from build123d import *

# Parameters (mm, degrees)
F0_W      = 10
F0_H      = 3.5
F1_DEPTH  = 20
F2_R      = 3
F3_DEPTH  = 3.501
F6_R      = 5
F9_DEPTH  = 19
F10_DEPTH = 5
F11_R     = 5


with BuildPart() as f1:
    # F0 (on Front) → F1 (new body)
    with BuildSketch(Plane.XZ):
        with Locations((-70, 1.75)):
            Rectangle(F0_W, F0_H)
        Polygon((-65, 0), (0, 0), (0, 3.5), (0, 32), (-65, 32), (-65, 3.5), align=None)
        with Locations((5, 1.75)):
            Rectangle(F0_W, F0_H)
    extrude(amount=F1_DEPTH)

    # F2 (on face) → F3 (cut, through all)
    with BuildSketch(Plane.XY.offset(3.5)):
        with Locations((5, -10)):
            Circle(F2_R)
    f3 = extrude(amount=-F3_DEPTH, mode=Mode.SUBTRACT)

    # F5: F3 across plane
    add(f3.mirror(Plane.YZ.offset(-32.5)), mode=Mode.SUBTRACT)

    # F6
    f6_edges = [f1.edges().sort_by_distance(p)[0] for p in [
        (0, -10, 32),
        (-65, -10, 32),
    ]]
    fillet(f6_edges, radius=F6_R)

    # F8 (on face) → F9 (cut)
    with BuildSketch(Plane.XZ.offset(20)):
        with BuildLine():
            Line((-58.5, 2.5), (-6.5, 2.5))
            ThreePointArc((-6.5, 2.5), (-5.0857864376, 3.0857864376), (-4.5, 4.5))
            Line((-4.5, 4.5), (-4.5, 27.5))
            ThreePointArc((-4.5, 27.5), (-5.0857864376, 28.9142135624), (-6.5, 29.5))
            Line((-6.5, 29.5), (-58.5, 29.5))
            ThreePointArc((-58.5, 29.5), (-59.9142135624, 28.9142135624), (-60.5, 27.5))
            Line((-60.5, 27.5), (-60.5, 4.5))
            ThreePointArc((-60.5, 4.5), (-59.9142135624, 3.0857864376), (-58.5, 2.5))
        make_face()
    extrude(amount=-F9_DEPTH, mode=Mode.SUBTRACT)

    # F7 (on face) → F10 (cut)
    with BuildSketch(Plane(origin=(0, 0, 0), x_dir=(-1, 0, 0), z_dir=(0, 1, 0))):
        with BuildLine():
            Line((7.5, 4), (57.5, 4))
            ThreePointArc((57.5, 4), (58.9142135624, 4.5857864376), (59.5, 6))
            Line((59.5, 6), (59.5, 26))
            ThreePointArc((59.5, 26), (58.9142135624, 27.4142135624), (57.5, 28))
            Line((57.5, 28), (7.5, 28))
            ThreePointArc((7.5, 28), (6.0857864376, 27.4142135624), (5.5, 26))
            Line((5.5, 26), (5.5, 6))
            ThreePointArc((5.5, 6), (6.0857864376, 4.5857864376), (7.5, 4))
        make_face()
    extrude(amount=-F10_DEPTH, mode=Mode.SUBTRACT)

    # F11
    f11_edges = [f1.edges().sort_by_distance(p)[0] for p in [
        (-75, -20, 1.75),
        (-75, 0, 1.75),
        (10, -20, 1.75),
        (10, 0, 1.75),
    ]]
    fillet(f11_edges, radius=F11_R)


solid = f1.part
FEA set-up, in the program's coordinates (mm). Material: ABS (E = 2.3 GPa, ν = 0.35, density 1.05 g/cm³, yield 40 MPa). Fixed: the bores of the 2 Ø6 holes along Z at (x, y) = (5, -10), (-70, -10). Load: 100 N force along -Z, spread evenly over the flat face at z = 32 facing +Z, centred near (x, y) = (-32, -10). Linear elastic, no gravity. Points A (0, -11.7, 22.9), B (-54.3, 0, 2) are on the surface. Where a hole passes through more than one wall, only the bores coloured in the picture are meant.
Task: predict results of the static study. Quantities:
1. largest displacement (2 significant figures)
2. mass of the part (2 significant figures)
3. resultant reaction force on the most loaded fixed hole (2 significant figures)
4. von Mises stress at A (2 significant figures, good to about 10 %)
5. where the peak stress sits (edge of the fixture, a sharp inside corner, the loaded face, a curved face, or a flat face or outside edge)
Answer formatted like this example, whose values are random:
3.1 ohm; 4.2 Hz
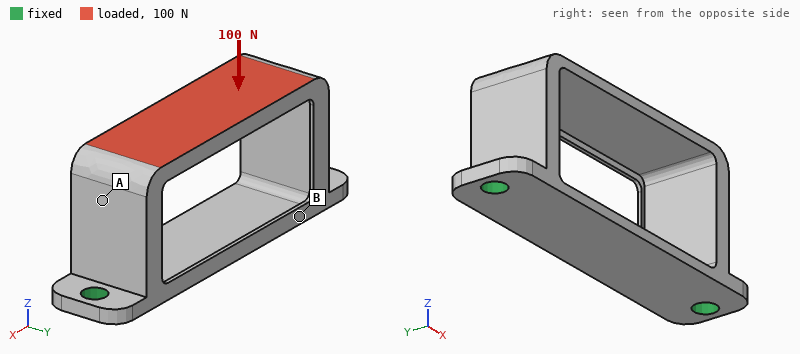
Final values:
0.94 mm; 13 g; 57 N; 3.8 MPa; a curved face
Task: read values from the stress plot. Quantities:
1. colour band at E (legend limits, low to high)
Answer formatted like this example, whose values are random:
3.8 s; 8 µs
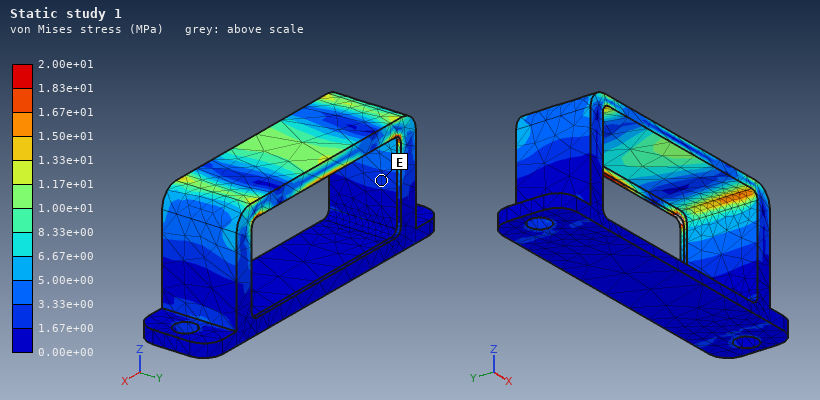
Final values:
1.67e+00 to 3.33e+00 MPa
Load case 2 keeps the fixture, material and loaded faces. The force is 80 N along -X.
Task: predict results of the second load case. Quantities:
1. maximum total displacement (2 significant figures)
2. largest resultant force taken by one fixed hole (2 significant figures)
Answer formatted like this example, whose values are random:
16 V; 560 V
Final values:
0.98 mm; 44 N
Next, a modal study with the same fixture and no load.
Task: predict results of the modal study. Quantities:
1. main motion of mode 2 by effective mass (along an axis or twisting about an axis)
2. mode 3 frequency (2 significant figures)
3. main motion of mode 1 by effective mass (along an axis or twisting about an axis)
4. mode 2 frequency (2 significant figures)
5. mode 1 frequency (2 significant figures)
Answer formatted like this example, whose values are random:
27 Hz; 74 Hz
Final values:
along Y; 1100 Hz; along X; 860 Hz; 660 Hz
